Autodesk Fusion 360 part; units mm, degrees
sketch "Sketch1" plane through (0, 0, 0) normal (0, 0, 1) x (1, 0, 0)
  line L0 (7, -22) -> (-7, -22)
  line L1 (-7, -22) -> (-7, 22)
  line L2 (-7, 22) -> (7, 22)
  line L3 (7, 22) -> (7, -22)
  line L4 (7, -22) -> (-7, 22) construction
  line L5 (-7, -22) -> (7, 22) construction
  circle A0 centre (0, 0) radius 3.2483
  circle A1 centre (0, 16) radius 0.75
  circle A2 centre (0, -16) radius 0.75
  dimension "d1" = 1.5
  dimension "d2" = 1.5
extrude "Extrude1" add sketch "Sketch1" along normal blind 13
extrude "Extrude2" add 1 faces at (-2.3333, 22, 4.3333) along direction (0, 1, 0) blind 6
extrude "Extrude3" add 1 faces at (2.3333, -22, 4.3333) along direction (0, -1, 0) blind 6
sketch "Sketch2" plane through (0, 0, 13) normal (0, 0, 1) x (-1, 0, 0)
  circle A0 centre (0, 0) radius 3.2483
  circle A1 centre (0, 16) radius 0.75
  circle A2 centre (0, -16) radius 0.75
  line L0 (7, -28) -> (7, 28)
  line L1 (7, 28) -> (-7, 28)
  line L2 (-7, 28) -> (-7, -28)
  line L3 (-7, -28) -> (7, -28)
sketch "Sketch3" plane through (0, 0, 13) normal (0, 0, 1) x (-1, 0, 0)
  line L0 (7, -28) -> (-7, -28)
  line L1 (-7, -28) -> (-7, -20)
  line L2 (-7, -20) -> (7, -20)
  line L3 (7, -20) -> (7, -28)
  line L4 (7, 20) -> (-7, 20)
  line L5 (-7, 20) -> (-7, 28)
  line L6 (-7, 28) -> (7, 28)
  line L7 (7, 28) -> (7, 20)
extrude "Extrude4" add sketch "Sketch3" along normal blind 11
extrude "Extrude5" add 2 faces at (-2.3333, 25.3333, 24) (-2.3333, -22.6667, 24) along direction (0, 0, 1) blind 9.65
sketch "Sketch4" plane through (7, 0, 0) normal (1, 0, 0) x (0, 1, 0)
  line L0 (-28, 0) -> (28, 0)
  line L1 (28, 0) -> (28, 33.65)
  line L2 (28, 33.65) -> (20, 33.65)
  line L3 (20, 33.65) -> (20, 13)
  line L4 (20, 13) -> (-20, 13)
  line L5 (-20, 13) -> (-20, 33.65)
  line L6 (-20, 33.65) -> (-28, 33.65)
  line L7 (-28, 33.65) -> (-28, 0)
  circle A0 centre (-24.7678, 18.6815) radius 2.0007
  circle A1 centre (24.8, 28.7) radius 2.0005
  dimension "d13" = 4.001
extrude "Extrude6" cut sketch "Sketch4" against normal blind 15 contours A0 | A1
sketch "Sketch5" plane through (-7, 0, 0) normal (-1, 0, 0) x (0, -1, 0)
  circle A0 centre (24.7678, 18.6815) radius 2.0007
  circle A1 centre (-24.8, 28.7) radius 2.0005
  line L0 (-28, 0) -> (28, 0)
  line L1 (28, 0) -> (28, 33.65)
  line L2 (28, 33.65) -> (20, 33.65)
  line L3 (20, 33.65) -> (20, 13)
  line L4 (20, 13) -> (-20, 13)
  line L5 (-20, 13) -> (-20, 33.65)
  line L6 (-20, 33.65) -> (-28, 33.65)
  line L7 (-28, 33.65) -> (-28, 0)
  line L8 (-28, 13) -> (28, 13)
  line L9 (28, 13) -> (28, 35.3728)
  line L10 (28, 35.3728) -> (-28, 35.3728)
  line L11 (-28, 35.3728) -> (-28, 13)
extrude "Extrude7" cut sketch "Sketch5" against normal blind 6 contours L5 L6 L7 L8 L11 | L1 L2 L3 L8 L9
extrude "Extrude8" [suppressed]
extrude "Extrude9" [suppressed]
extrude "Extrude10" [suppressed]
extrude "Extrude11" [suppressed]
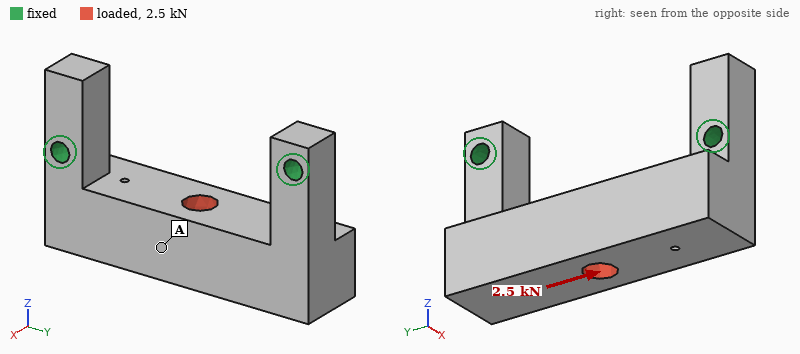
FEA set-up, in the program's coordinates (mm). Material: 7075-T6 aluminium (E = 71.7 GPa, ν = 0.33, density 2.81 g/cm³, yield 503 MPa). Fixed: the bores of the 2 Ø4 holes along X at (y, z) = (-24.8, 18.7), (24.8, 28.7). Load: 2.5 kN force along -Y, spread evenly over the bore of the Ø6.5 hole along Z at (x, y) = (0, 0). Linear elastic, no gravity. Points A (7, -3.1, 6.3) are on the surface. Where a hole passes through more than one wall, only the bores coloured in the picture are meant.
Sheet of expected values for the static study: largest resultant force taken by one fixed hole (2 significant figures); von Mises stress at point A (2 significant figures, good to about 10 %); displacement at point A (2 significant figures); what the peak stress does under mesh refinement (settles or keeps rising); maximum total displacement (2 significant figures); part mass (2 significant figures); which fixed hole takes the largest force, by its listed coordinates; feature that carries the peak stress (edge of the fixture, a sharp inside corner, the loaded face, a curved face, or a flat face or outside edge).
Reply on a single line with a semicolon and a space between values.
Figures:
1.9 kN; 14 MPa; 22 µm; keeps rising; 26 µm; 34 g; (-24.8, 18.7); edge of the fixture
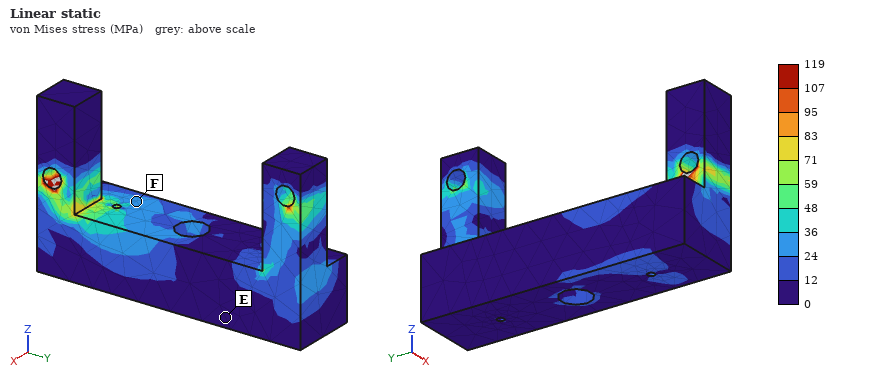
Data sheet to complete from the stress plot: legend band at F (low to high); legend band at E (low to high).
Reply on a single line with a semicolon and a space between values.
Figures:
24 to 36 MPa; 0 to 12 MPa
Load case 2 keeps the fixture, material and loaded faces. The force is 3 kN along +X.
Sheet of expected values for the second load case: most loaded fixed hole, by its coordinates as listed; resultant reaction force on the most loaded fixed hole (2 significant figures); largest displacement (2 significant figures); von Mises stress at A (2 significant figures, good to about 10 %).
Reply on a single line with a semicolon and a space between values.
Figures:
(-24.8, 18.7); 1.7 kN; 0.20 mm; 68 MPa
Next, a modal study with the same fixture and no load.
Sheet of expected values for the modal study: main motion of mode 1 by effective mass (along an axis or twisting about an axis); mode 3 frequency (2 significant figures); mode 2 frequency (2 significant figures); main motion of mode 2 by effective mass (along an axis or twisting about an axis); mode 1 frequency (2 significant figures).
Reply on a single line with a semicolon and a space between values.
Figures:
along X; 12 kHz; 9900 Hz; along Y; 4500 Hz
